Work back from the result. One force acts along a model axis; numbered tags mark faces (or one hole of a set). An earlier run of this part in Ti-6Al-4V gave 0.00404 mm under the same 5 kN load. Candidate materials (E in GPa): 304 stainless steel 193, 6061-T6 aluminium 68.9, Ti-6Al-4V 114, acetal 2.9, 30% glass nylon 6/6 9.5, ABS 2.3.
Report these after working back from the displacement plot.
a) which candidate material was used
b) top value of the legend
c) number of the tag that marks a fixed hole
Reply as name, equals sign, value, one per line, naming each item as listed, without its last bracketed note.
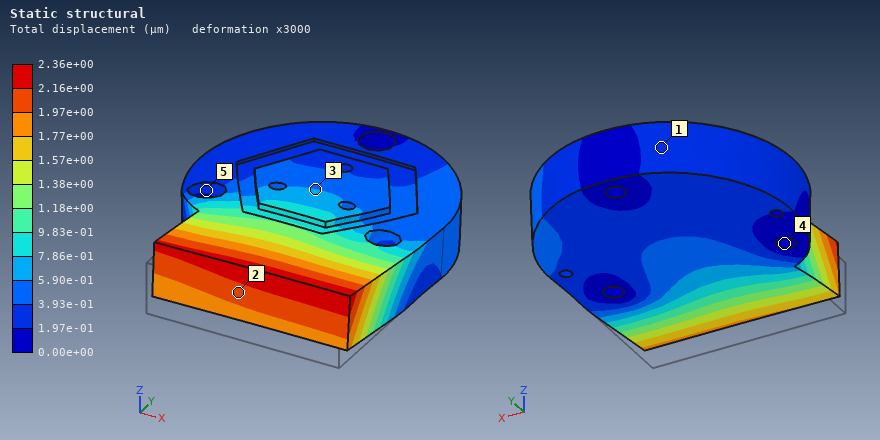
which candidate material was used = 304 stainless steel
top value of the legend = 2.36e+00 µm
number of the tag that marks a fixed hole = 4
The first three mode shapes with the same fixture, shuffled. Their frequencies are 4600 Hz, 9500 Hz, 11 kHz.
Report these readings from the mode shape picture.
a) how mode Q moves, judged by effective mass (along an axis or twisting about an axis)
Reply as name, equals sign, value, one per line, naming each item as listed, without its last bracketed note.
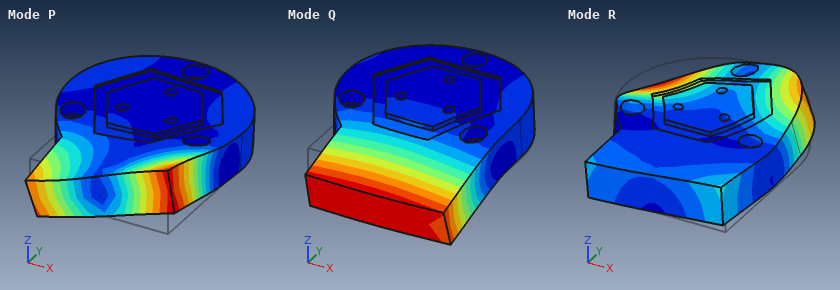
how mode Q moves, judged by effective mass = along Z
